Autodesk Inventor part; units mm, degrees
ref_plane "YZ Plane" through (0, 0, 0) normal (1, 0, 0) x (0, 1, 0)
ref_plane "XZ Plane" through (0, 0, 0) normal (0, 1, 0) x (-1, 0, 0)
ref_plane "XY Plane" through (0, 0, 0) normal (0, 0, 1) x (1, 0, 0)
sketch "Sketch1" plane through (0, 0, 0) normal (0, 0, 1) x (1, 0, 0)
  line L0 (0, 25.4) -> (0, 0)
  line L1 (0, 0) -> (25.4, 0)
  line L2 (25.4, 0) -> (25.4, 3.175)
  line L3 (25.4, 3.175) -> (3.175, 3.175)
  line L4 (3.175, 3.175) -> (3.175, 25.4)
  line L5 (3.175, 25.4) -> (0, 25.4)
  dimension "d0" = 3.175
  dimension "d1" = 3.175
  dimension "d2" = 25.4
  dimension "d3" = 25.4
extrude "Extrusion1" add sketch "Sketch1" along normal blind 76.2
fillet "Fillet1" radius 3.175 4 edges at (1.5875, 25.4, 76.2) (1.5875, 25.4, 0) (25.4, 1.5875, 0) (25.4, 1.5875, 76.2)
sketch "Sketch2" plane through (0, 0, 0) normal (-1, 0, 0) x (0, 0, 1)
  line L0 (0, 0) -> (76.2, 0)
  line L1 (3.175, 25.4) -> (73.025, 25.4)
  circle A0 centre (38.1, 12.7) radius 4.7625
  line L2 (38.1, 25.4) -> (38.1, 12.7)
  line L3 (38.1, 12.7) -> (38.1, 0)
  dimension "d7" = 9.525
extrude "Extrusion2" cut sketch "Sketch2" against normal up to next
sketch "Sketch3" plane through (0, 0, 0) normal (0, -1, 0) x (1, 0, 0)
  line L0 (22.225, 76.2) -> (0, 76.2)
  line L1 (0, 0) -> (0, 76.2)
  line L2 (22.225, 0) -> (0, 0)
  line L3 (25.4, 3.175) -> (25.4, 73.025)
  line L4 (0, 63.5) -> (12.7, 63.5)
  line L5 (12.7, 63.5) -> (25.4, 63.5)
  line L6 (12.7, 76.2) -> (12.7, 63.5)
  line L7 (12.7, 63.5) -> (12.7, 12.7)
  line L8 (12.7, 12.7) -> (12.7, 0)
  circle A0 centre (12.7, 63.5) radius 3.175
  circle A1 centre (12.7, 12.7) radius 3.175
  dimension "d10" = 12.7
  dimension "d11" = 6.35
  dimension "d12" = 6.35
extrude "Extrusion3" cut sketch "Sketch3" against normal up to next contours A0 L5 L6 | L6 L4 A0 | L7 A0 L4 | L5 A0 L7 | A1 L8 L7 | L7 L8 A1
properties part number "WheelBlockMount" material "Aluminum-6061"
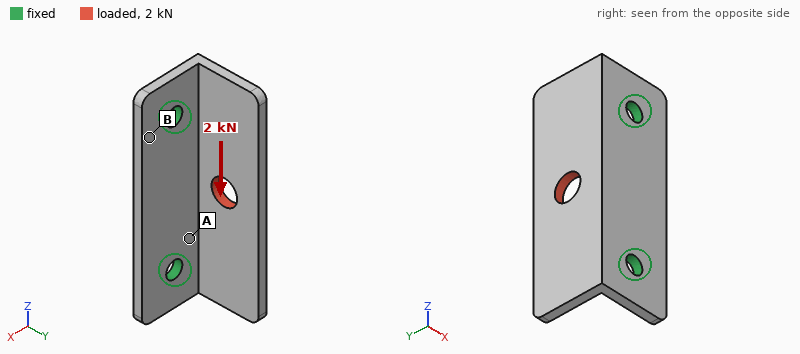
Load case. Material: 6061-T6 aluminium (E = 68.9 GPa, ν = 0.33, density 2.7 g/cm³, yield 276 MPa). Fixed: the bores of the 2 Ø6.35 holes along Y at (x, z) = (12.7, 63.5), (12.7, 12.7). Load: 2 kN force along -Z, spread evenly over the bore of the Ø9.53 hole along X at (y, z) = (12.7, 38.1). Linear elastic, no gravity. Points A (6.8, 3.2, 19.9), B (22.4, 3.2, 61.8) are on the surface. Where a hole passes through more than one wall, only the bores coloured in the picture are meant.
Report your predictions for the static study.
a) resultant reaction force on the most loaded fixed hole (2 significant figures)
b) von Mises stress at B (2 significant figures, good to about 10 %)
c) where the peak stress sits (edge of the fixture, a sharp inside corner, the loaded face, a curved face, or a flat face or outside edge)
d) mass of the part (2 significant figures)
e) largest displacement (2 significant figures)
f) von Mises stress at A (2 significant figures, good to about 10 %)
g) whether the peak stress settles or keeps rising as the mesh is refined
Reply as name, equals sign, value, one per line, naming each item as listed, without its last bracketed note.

resultant reaction force on the most loaded fixed hole = 1.1 kN
von Mises stress at B = 8.6 MPa
where the peak stress sits = edge of the fixture
mass of the part = 30 g
largest displacement = 75 µm
von Mises stress at A = 42 MPa
whether the peak stress settles or keeps rising as the mesh is refined = keeps rising
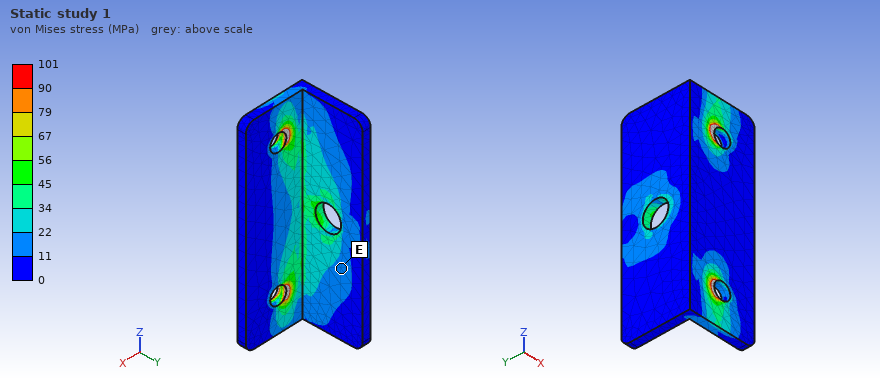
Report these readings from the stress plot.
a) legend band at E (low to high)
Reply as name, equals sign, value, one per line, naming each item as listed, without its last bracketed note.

legend band at E = 11 to 22 MPa
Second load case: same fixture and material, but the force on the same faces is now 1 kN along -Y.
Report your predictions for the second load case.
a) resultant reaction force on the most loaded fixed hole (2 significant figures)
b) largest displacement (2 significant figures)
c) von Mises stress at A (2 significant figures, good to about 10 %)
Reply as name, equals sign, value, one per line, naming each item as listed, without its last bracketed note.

resultant reaction force on the most loaded fixed hole = 540 N
largest displacement = 0.12 mm
von Mises stress at A = 38 MPa
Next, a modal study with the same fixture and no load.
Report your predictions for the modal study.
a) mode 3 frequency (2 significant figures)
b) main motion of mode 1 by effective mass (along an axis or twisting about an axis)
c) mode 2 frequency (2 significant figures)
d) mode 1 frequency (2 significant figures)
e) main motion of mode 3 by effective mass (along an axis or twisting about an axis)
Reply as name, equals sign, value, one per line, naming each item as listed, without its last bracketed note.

mode 3 frequency = 7000 Hz
main motion of mode 1 by effective mass = along X
mode 2 frequency = 3900 Hz
mode 1 frequency = 2700 Hz
main motion of mode 3 by effective mass = along Y
